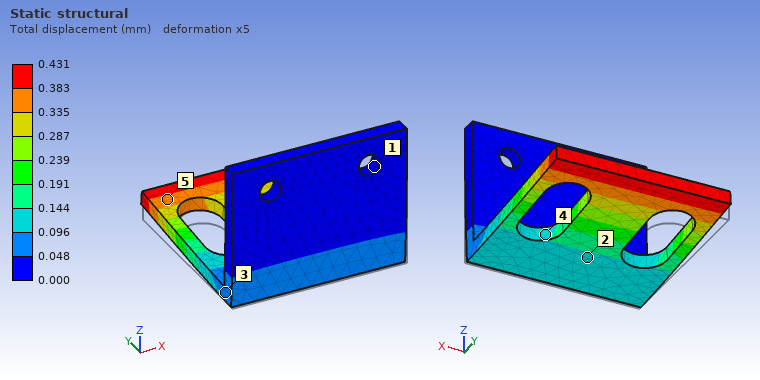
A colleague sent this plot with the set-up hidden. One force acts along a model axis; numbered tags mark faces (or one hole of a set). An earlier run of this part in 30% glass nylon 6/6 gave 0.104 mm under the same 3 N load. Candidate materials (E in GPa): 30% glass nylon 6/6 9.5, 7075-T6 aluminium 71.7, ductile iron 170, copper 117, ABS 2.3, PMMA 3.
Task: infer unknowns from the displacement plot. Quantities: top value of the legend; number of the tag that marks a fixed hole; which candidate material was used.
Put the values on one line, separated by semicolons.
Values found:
0.431 mm; 1; ABS
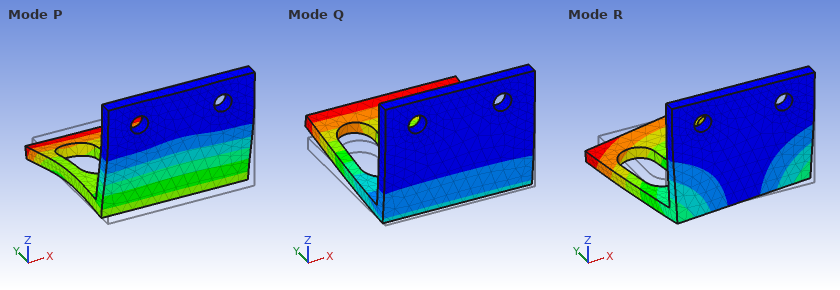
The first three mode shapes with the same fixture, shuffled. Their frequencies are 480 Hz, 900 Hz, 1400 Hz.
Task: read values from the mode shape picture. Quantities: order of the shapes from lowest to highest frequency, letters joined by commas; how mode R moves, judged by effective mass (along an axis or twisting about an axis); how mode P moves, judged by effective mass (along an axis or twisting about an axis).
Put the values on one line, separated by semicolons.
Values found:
Q, R, P; along X; along Y
